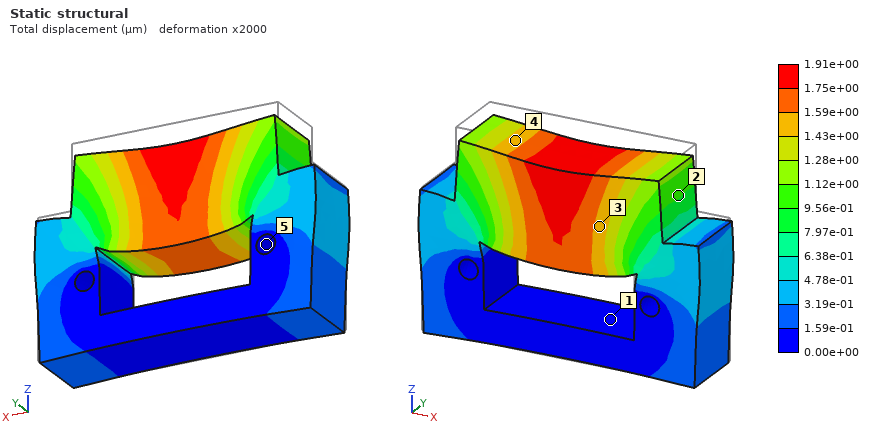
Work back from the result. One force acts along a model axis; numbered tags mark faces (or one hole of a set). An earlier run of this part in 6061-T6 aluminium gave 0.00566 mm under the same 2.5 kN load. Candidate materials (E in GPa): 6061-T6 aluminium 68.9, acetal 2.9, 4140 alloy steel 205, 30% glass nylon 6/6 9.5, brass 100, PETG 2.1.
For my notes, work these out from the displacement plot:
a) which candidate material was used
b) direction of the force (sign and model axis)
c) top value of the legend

4140 alloy steel
-Z
1.91e+00 µm
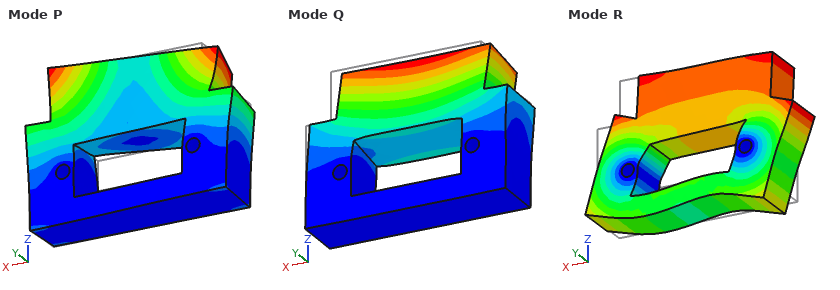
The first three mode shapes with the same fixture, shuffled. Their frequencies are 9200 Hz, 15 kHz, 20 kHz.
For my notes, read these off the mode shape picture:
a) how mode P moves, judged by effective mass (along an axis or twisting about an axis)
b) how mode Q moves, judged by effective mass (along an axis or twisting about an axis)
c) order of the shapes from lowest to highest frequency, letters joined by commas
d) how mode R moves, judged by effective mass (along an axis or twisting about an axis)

twisting about Z
along Y
Q, R, P
along X
